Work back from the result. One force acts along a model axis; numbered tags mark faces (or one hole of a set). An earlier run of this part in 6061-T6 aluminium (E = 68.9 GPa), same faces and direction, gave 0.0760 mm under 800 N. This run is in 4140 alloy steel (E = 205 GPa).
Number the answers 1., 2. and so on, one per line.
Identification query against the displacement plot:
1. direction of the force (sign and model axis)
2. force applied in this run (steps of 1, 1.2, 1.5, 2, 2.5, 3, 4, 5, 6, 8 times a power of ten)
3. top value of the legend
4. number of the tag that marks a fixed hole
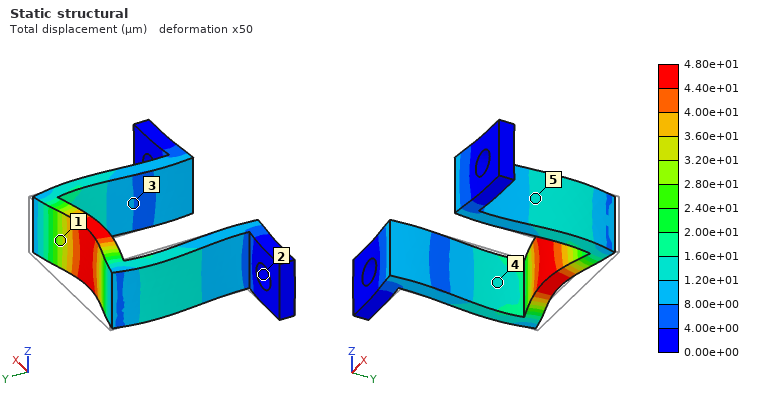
1. -Y
2. 1.5 kN
3. 4.80e+01 µm
4. 2
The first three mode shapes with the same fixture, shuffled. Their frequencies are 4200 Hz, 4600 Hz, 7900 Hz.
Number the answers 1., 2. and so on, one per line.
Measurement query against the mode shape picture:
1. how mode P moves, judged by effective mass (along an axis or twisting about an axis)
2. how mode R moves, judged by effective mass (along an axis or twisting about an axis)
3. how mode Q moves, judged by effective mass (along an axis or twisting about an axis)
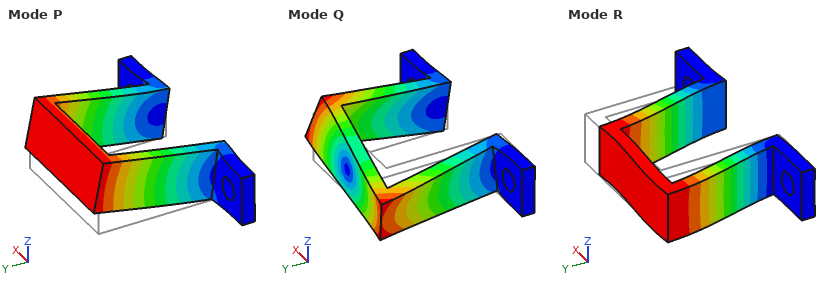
1. along Z
2. along X
3. twisting about Y
